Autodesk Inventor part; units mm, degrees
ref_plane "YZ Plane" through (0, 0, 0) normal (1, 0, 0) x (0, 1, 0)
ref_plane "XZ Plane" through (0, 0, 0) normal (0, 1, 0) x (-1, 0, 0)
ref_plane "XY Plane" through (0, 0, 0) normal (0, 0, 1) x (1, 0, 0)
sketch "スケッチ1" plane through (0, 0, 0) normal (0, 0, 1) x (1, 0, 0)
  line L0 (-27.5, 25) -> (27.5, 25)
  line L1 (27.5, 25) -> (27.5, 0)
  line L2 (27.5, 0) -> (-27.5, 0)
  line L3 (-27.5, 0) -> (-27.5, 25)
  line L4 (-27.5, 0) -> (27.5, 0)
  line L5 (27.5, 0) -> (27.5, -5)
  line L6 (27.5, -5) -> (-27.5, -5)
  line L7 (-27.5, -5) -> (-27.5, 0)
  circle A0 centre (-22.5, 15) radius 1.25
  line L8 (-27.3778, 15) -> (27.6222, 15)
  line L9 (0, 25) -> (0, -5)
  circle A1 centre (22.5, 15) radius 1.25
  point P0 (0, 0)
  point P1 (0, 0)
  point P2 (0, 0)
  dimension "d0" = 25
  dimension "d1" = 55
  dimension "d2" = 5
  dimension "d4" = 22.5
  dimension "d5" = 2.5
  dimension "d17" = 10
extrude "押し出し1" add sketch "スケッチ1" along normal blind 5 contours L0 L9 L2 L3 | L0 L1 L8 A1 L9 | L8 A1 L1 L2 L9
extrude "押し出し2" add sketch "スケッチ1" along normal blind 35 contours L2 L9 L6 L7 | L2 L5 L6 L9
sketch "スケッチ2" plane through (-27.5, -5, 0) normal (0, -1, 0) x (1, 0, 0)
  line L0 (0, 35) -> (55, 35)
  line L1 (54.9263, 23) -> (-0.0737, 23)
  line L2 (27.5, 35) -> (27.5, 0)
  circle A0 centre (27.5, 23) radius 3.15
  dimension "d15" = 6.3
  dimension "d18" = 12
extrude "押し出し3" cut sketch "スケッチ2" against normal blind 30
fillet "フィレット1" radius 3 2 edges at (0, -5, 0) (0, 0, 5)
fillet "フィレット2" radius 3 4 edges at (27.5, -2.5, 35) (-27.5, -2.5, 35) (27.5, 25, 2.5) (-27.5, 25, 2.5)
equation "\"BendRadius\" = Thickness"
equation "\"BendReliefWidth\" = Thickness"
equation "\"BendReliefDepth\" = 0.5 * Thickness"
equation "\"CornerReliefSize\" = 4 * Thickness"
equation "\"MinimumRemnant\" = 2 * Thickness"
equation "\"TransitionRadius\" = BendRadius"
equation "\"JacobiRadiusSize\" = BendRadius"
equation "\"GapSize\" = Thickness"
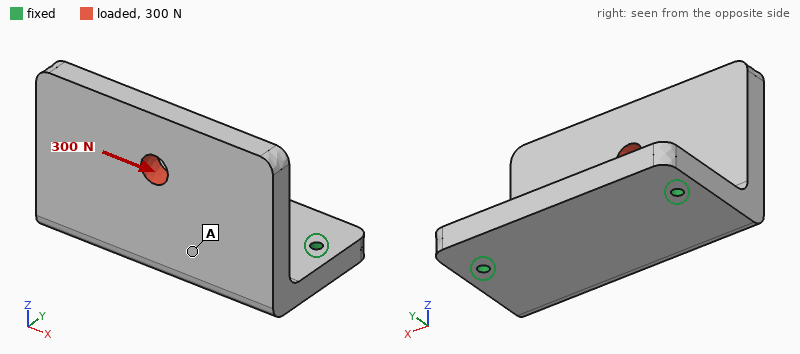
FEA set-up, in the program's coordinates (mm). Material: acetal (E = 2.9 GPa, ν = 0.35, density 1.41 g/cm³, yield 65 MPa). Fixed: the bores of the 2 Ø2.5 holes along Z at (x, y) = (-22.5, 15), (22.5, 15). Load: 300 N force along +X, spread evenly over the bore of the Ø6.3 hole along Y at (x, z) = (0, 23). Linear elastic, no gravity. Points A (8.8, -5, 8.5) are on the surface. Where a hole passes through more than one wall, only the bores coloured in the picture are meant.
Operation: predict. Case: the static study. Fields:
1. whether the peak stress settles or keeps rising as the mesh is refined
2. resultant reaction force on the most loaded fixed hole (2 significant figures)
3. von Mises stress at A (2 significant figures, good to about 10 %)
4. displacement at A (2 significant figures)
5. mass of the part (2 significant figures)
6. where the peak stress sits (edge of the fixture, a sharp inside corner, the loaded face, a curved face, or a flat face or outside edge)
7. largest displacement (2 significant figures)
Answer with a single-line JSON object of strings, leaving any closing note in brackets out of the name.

{"whether the peak stress settles or keeps rising as the mesh is refined": "keeps rising", "resultant reaction force on the most loaded fixed hole": "230 N", "von Mises stress at A": "3.3 MPa", "displacement at A": "0.14 mm", "mass of the part": "23 g", "where the peak stress sits": "edge of the fixture", "largest displacement": "0.59 mm"}
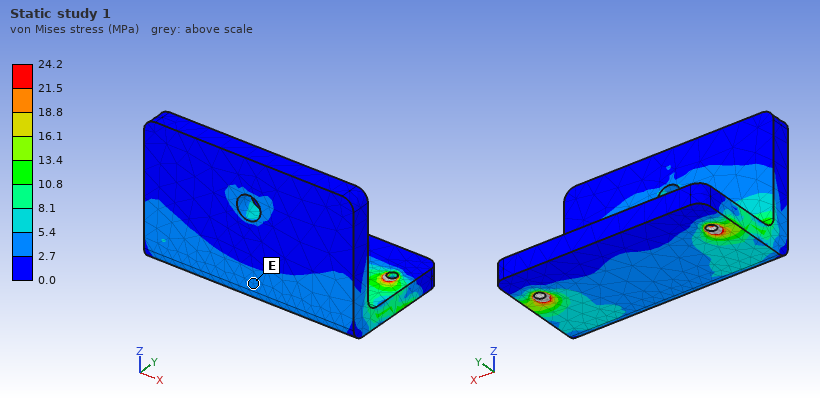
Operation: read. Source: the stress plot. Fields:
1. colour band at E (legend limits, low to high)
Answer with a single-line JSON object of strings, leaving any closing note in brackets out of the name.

{"colour band at E": "2.7 to 5.4 MPa"}
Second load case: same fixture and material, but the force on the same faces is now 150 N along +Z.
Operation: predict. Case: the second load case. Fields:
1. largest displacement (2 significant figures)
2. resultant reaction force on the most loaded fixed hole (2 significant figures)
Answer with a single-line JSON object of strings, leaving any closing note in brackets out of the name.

{"largest displacement": "0.81 mm", "resultant reaction force on the most loaded fixed hole": "75 N"}
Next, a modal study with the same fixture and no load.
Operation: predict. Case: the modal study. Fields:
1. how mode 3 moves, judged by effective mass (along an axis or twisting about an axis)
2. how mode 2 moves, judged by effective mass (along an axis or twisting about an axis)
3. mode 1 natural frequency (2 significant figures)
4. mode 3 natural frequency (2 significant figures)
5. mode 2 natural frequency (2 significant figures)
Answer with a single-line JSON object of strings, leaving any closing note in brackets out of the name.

{"how mode 3 moves, judged by effective mass": "along Z", "how mode 2 moves, judged by effective mass": "along X", "mode 1 natural frequency": "530 Hz", "mode 3 natural frequency": "1600 Hz", "mode 2 natural frequency": "1100 Hz"}
